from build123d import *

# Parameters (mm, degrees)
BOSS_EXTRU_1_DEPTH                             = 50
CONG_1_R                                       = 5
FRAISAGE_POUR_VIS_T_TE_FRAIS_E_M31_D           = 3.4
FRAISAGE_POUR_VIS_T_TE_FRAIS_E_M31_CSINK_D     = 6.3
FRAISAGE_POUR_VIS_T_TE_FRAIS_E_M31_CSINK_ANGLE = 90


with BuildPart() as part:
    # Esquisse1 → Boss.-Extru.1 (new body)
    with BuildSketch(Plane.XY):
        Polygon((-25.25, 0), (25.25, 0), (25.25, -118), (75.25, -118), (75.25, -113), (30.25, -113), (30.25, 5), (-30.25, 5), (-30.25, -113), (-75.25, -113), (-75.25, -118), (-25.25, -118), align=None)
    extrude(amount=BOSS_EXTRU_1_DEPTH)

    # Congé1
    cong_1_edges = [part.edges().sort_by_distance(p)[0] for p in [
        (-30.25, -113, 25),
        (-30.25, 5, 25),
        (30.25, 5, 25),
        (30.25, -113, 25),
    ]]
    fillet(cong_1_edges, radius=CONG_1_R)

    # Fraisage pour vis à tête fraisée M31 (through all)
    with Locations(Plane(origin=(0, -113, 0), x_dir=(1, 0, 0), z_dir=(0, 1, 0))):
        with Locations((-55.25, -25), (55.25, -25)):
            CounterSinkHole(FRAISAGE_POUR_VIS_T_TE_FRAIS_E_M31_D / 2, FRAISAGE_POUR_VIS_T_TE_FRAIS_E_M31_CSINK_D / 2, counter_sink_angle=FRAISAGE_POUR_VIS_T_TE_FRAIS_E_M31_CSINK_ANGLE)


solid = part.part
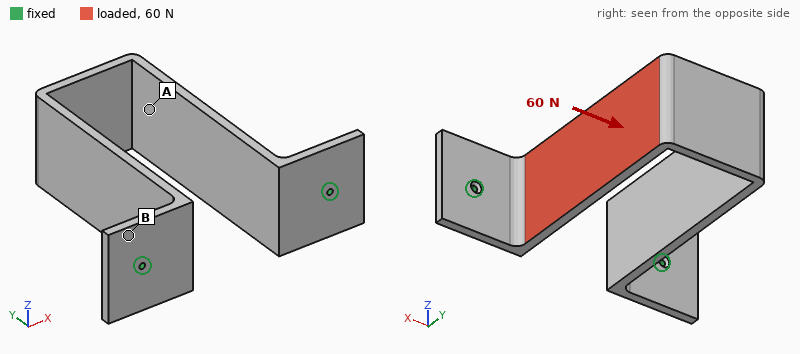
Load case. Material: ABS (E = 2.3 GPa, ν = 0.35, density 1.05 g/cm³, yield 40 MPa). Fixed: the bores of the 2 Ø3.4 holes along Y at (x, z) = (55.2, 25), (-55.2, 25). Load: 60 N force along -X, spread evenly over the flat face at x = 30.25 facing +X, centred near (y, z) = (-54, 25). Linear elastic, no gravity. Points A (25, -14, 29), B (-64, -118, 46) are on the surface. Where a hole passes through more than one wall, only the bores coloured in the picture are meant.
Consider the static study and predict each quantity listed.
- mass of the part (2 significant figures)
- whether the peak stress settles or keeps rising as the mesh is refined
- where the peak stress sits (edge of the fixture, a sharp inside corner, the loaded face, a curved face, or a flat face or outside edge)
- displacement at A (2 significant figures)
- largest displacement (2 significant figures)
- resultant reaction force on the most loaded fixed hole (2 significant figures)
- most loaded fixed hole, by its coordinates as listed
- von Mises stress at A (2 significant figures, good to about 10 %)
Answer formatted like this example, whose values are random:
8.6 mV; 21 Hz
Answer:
100 g; keeps rising; edge of the fixture; 2.3 mm; 2.4 mm; 52 N; (55.2, 25); 3.4 MPa
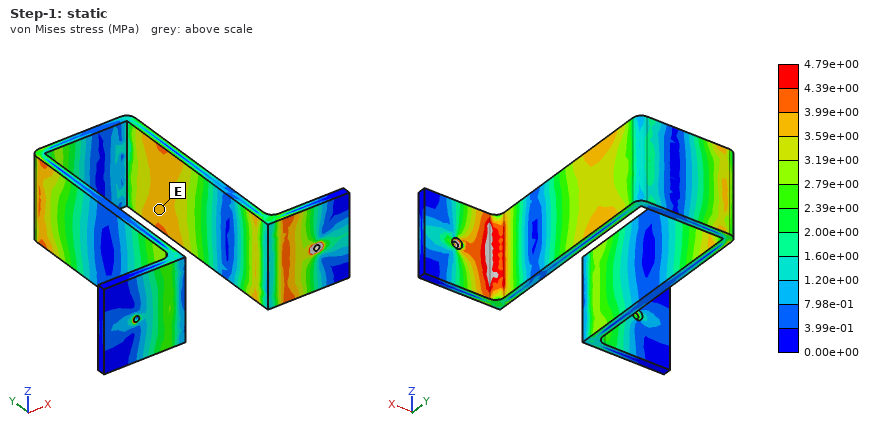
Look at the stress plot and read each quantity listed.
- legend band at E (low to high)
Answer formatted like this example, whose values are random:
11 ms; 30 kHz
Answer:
3.59e+00 to 3.99e+00 MPa
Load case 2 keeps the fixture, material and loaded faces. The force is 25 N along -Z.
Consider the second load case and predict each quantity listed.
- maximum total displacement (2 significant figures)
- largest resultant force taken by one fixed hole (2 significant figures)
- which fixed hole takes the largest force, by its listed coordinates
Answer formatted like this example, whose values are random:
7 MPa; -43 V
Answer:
2.3 mm; 20 N; (55.2, 25)
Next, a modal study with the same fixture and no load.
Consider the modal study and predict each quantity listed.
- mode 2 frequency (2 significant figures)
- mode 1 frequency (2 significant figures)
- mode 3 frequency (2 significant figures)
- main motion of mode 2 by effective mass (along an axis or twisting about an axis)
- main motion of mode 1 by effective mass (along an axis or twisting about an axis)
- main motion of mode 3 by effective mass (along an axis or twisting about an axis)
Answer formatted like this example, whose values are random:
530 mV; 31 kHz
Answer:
97 Hz; 68 Hz; 210 Hz; along X; along Z; twisting about Y
